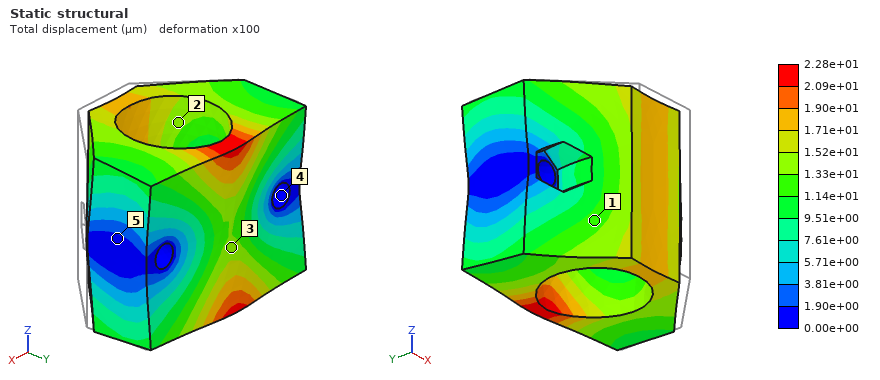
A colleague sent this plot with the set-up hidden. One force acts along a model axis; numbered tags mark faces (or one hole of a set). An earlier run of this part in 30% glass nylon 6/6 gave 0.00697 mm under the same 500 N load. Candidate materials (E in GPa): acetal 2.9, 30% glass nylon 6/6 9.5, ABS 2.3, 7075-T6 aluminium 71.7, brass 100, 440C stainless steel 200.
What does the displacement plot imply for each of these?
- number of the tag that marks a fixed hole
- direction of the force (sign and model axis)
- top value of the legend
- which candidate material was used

4
+Y
2.28e+01 µm
acetal
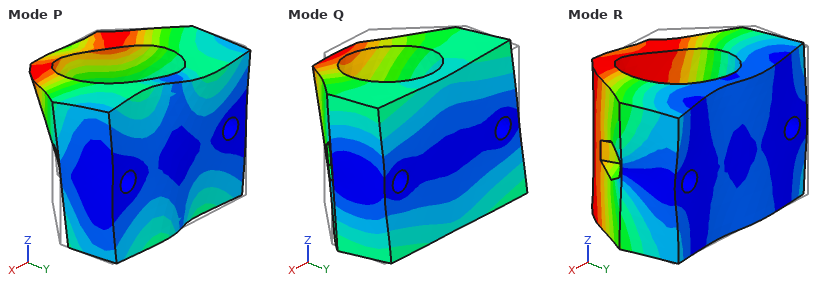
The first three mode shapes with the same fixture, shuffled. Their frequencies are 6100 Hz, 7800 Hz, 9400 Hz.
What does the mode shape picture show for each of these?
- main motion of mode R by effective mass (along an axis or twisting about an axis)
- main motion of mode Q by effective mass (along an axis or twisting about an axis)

along X
along Z
